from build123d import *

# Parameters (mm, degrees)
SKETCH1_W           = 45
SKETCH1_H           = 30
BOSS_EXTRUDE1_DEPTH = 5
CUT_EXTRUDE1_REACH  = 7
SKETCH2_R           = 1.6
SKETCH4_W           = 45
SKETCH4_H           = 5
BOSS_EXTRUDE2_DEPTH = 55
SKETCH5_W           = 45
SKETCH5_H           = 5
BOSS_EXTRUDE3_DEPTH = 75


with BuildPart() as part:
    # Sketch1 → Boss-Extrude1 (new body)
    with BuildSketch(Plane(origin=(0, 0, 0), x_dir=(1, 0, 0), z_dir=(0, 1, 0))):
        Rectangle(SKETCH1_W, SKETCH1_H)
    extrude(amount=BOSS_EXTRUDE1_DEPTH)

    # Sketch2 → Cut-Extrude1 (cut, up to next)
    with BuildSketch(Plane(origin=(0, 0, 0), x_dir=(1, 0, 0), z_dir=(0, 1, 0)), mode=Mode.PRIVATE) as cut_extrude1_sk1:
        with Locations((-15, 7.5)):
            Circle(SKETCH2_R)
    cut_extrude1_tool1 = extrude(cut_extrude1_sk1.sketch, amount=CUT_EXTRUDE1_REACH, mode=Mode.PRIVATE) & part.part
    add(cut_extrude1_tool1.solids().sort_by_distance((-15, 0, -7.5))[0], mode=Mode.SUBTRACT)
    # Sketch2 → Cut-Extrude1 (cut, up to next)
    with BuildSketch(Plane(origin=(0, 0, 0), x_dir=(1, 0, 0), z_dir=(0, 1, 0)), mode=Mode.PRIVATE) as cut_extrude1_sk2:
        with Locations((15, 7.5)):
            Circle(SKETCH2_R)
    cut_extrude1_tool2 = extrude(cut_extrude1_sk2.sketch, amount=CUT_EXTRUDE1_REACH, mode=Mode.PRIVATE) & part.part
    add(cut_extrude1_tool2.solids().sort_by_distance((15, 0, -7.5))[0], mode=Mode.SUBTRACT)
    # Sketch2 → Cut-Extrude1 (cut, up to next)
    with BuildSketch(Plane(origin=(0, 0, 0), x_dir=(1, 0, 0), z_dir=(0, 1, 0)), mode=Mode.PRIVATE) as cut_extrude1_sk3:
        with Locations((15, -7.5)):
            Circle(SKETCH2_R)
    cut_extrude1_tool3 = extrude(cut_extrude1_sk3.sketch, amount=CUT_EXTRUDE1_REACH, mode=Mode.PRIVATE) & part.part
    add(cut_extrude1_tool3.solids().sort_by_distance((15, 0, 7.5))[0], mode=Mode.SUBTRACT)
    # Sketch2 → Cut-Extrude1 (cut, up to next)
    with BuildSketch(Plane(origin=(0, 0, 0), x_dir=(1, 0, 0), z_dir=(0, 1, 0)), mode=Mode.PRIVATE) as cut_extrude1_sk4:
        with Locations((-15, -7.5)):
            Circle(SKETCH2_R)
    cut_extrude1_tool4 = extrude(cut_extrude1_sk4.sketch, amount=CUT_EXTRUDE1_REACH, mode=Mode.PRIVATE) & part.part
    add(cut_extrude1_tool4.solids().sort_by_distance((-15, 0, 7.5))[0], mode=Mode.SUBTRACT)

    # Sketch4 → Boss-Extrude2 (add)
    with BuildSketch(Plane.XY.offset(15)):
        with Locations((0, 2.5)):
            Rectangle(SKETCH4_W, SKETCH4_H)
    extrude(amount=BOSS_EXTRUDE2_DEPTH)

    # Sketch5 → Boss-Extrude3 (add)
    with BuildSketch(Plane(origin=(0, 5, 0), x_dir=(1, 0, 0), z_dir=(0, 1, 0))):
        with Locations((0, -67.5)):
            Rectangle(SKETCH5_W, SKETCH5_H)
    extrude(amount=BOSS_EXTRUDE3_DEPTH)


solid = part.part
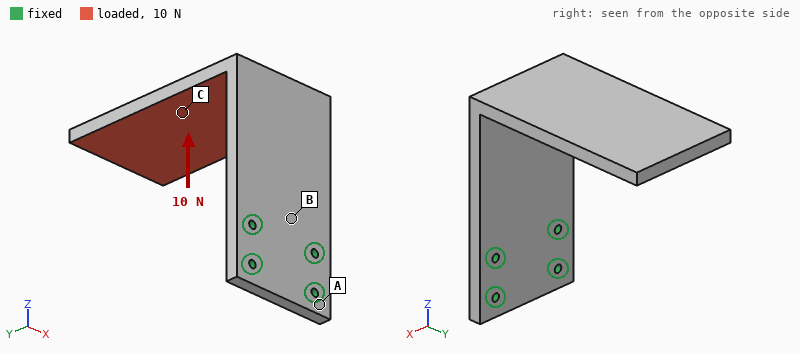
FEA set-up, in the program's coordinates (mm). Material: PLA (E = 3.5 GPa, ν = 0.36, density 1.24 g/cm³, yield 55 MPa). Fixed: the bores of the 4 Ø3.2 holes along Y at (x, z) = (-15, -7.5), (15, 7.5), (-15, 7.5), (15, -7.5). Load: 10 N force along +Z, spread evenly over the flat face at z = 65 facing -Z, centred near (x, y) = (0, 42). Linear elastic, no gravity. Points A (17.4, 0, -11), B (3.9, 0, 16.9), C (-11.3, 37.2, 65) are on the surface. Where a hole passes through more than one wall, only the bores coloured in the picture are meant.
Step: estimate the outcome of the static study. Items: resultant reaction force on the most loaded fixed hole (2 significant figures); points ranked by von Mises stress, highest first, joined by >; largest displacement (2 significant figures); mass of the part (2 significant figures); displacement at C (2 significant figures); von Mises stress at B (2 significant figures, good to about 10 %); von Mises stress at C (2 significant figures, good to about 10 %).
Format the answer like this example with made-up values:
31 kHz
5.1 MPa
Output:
6.8 N
B > C > A
1.5 mm
44 g
0.70 mm
1.8 MPa
0.64 MPa
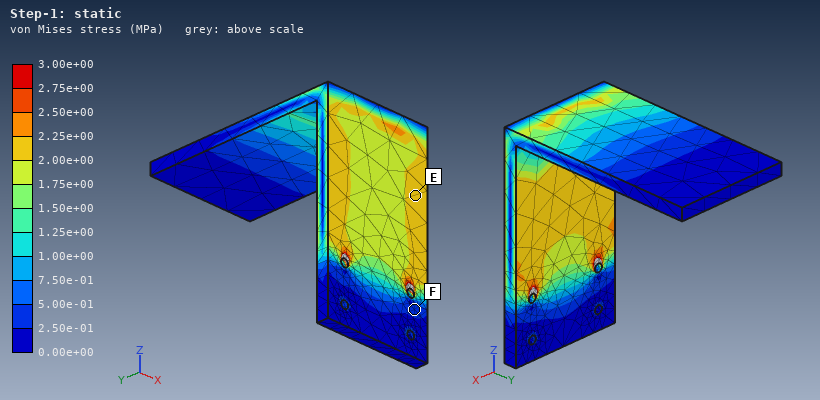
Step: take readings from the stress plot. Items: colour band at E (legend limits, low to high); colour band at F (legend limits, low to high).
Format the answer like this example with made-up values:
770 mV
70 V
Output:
2.00e+00 to 2.25e+00 MPa
2.50e-01 to 5.00e-01 MPa
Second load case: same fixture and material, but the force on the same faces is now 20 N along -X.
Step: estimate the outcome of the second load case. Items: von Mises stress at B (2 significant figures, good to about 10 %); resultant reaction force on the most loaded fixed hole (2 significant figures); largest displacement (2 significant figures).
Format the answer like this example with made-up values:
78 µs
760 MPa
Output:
2.1 MPa
43 N
1.3 mm
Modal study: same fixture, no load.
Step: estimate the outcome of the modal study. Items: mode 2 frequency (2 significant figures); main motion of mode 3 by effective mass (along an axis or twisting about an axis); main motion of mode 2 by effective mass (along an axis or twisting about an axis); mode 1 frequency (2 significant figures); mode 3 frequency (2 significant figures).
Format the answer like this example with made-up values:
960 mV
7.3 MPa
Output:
160 Hz
along Y
along X
96 Hz
270 Hz
